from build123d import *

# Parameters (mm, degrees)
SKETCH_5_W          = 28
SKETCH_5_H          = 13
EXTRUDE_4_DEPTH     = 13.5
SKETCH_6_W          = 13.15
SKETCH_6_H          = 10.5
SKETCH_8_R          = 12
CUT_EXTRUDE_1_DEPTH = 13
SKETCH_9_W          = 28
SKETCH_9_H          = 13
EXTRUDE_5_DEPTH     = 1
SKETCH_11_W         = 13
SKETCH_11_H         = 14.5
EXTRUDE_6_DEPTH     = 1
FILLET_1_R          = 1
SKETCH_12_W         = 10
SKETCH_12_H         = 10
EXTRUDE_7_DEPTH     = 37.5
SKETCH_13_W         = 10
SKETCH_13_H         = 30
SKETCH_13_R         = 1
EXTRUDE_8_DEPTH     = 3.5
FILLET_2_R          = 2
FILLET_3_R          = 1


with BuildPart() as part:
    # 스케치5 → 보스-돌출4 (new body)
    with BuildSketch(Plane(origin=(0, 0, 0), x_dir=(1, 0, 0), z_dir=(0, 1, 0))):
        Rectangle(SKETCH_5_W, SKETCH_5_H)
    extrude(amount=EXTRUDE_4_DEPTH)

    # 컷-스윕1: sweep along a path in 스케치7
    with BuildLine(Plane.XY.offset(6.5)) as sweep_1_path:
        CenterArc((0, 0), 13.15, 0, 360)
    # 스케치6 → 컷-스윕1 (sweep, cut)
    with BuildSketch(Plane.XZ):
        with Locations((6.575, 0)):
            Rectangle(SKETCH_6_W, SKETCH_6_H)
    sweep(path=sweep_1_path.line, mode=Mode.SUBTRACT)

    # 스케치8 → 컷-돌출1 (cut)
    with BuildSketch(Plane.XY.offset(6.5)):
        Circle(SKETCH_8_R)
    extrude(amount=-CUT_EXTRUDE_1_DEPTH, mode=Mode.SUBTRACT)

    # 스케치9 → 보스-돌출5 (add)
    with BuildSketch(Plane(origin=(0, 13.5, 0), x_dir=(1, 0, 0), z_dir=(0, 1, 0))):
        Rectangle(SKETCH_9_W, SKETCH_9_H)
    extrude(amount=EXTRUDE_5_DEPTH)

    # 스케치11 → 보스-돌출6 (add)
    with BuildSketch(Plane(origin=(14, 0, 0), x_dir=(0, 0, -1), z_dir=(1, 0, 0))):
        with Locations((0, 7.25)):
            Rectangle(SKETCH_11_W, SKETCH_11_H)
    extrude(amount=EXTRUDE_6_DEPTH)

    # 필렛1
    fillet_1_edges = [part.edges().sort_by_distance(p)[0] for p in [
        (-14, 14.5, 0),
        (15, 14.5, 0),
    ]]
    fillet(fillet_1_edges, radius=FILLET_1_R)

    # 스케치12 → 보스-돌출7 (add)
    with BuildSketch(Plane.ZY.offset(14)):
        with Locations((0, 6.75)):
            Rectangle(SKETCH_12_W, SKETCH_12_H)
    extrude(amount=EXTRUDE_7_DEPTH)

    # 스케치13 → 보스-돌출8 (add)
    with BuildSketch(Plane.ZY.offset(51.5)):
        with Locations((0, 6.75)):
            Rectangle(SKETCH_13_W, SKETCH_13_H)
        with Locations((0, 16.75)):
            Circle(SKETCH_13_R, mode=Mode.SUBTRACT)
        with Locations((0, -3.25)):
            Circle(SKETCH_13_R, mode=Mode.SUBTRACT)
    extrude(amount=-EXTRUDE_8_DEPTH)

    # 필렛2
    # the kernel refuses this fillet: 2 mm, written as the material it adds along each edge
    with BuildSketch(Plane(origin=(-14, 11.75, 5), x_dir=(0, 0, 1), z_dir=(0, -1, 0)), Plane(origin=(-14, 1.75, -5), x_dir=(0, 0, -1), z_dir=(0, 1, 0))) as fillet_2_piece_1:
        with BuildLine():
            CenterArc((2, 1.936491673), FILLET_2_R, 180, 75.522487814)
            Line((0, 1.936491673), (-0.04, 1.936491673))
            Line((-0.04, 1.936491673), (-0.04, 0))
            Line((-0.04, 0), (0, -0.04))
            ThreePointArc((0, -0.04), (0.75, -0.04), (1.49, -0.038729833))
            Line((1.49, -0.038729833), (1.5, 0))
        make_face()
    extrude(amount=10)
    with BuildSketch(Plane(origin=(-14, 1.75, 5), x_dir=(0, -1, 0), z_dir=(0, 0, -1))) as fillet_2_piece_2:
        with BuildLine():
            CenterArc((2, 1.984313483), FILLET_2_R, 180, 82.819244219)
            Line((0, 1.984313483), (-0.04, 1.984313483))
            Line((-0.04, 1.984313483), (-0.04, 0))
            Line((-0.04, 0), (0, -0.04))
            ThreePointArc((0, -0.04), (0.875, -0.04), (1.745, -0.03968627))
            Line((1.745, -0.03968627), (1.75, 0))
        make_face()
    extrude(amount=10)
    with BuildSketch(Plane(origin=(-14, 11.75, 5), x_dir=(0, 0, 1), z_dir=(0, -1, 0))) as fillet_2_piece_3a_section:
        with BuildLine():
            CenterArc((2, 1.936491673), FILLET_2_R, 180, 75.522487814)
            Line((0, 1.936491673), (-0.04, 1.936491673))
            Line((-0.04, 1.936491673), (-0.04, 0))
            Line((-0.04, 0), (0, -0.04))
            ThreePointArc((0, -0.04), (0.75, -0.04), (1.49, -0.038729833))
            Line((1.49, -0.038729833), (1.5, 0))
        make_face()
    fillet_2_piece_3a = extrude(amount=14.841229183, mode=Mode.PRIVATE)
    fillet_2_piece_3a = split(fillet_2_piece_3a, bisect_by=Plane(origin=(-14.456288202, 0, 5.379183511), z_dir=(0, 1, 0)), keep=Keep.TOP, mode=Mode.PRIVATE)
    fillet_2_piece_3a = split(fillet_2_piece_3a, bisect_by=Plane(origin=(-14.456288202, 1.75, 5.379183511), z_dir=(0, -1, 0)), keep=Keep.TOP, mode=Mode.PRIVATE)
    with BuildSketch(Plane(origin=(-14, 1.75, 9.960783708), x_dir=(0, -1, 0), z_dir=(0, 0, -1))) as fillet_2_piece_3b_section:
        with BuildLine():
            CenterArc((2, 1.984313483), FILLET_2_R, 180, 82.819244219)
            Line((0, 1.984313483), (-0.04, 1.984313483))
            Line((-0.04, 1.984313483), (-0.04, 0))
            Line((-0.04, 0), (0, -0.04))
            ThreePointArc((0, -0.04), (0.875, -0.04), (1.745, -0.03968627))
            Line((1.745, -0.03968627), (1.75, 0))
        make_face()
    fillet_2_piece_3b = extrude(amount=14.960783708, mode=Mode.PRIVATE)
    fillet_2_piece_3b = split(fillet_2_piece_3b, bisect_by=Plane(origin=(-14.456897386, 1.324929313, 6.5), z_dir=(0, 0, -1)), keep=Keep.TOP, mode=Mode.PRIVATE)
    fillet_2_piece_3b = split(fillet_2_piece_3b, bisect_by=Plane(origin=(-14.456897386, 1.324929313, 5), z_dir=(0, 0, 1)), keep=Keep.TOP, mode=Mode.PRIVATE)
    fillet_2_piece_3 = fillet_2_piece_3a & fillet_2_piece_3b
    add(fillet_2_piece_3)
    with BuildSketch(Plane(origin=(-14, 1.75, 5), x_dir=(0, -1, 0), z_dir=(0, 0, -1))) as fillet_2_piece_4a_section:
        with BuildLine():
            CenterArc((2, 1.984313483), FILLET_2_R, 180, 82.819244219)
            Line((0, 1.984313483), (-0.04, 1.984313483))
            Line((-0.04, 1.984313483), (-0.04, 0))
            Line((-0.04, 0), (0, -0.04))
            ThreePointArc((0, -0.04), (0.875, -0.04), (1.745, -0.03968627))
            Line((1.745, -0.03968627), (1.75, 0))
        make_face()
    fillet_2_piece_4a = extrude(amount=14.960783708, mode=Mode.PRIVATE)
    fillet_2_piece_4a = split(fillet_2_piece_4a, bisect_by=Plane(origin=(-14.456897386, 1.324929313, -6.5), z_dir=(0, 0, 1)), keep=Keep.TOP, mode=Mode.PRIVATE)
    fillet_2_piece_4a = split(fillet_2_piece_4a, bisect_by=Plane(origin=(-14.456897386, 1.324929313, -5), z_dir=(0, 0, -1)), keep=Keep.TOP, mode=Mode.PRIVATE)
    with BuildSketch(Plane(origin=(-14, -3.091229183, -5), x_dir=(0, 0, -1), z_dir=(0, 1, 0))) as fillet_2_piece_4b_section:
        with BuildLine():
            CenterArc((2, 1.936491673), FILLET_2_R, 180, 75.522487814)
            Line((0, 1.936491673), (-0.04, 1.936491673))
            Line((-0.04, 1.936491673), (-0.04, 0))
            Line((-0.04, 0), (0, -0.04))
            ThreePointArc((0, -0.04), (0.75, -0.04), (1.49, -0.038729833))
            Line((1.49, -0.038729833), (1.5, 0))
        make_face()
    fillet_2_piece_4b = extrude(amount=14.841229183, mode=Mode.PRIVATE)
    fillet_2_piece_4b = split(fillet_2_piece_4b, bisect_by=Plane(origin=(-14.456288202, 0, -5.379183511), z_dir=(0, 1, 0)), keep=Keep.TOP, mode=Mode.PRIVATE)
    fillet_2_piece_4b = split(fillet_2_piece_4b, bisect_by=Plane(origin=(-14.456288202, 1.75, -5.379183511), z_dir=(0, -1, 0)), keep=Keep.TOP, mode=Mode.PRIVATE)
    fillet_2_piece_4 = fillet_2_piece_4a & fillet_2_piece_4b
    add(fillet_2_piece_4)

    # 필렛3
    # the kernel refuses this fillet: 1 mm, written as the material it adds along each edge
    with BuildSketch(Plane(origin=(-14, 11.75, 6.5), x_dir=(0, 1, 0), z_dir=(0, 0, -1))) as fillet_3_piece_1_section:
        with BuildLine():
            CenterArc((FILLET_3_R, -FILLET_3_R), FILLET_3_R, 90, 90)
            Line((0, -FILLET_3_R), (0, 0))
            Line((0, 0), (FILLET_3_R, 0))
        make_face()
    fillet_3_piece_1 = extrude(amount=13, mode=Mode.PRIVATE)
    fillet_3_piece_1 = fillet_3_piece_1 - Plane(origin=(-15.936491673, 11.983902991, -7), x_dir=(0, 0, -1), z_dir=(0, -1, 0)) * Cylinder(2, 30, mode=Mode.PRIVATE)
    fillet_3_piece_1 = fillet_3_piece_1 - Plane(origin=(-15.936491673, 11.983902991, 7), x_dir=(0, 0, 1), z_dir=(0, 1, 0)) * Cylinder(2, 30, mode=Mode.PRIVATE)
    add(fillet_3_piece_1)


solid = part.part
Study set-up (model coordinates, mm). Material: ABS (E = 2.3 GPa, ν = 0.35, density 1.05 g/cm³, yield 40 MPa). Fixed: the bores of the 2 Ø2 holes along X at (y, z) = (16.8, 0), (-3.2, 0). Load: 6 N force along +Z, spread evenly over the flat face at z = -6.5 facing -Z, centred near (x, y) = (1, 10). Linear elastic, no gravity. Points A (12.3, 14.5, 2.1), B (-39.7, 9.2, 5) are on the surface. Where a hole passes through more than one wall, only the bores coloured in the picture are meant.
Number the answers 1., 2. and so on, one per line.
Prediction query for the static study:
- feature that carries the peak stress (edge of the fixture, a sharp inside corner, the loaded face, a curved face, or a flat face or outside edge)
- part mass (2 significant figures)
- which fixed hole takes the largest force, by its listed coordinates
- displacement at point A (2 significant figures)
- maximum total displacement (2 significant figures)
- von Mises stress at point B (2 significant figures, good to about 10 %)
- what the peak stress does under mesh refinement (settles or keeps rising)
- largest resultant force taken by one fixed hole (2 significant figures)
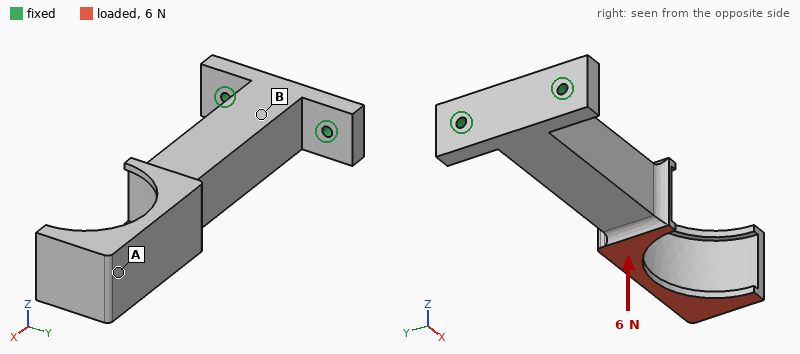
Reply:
1. edge of the fixture
2. 6.8 g
3. (16.8, 0)
4. 0.71 mm
5. 0.81 mm
6. 1.5 MPa
7. keeps rising
8. 3.9 N
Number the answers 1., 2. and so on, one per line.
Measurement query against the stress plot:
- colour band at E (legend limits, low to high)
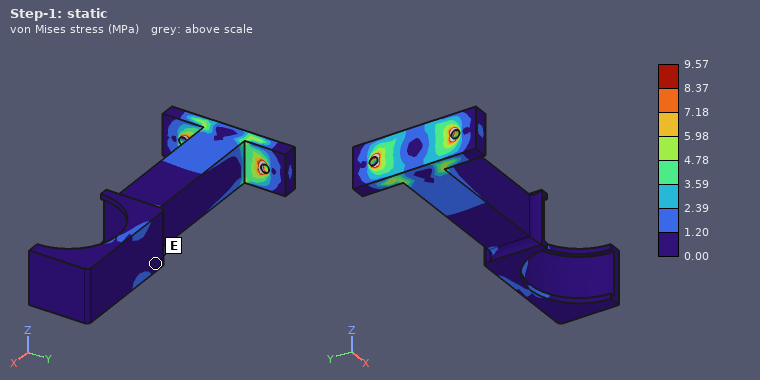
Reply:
1. 0.00 to 1.20 MPa
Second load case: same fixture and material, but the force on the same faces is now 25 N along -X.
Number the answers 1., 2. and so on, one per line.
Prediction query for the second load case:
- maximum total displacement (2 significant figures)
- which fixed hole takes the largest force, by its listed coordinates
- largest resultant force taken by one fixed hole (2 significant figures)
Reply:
1. 0.74 mm
2. (16.8, 0)
3. 18 N
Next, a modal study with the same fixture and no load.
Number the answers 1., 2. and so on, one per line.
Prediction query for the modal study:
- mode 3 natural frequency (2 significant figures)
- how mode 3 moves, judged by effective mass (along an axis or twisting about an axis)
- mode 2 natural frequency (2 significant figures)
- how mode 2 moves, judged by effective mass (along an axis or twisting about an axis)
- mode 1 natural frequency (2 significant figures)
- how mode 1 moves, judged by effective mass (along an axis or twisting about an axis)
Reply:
1. 940 Hz
2. along Y
3. 380 Hz
4. along Y
5. 300 Hz
6. along Z
